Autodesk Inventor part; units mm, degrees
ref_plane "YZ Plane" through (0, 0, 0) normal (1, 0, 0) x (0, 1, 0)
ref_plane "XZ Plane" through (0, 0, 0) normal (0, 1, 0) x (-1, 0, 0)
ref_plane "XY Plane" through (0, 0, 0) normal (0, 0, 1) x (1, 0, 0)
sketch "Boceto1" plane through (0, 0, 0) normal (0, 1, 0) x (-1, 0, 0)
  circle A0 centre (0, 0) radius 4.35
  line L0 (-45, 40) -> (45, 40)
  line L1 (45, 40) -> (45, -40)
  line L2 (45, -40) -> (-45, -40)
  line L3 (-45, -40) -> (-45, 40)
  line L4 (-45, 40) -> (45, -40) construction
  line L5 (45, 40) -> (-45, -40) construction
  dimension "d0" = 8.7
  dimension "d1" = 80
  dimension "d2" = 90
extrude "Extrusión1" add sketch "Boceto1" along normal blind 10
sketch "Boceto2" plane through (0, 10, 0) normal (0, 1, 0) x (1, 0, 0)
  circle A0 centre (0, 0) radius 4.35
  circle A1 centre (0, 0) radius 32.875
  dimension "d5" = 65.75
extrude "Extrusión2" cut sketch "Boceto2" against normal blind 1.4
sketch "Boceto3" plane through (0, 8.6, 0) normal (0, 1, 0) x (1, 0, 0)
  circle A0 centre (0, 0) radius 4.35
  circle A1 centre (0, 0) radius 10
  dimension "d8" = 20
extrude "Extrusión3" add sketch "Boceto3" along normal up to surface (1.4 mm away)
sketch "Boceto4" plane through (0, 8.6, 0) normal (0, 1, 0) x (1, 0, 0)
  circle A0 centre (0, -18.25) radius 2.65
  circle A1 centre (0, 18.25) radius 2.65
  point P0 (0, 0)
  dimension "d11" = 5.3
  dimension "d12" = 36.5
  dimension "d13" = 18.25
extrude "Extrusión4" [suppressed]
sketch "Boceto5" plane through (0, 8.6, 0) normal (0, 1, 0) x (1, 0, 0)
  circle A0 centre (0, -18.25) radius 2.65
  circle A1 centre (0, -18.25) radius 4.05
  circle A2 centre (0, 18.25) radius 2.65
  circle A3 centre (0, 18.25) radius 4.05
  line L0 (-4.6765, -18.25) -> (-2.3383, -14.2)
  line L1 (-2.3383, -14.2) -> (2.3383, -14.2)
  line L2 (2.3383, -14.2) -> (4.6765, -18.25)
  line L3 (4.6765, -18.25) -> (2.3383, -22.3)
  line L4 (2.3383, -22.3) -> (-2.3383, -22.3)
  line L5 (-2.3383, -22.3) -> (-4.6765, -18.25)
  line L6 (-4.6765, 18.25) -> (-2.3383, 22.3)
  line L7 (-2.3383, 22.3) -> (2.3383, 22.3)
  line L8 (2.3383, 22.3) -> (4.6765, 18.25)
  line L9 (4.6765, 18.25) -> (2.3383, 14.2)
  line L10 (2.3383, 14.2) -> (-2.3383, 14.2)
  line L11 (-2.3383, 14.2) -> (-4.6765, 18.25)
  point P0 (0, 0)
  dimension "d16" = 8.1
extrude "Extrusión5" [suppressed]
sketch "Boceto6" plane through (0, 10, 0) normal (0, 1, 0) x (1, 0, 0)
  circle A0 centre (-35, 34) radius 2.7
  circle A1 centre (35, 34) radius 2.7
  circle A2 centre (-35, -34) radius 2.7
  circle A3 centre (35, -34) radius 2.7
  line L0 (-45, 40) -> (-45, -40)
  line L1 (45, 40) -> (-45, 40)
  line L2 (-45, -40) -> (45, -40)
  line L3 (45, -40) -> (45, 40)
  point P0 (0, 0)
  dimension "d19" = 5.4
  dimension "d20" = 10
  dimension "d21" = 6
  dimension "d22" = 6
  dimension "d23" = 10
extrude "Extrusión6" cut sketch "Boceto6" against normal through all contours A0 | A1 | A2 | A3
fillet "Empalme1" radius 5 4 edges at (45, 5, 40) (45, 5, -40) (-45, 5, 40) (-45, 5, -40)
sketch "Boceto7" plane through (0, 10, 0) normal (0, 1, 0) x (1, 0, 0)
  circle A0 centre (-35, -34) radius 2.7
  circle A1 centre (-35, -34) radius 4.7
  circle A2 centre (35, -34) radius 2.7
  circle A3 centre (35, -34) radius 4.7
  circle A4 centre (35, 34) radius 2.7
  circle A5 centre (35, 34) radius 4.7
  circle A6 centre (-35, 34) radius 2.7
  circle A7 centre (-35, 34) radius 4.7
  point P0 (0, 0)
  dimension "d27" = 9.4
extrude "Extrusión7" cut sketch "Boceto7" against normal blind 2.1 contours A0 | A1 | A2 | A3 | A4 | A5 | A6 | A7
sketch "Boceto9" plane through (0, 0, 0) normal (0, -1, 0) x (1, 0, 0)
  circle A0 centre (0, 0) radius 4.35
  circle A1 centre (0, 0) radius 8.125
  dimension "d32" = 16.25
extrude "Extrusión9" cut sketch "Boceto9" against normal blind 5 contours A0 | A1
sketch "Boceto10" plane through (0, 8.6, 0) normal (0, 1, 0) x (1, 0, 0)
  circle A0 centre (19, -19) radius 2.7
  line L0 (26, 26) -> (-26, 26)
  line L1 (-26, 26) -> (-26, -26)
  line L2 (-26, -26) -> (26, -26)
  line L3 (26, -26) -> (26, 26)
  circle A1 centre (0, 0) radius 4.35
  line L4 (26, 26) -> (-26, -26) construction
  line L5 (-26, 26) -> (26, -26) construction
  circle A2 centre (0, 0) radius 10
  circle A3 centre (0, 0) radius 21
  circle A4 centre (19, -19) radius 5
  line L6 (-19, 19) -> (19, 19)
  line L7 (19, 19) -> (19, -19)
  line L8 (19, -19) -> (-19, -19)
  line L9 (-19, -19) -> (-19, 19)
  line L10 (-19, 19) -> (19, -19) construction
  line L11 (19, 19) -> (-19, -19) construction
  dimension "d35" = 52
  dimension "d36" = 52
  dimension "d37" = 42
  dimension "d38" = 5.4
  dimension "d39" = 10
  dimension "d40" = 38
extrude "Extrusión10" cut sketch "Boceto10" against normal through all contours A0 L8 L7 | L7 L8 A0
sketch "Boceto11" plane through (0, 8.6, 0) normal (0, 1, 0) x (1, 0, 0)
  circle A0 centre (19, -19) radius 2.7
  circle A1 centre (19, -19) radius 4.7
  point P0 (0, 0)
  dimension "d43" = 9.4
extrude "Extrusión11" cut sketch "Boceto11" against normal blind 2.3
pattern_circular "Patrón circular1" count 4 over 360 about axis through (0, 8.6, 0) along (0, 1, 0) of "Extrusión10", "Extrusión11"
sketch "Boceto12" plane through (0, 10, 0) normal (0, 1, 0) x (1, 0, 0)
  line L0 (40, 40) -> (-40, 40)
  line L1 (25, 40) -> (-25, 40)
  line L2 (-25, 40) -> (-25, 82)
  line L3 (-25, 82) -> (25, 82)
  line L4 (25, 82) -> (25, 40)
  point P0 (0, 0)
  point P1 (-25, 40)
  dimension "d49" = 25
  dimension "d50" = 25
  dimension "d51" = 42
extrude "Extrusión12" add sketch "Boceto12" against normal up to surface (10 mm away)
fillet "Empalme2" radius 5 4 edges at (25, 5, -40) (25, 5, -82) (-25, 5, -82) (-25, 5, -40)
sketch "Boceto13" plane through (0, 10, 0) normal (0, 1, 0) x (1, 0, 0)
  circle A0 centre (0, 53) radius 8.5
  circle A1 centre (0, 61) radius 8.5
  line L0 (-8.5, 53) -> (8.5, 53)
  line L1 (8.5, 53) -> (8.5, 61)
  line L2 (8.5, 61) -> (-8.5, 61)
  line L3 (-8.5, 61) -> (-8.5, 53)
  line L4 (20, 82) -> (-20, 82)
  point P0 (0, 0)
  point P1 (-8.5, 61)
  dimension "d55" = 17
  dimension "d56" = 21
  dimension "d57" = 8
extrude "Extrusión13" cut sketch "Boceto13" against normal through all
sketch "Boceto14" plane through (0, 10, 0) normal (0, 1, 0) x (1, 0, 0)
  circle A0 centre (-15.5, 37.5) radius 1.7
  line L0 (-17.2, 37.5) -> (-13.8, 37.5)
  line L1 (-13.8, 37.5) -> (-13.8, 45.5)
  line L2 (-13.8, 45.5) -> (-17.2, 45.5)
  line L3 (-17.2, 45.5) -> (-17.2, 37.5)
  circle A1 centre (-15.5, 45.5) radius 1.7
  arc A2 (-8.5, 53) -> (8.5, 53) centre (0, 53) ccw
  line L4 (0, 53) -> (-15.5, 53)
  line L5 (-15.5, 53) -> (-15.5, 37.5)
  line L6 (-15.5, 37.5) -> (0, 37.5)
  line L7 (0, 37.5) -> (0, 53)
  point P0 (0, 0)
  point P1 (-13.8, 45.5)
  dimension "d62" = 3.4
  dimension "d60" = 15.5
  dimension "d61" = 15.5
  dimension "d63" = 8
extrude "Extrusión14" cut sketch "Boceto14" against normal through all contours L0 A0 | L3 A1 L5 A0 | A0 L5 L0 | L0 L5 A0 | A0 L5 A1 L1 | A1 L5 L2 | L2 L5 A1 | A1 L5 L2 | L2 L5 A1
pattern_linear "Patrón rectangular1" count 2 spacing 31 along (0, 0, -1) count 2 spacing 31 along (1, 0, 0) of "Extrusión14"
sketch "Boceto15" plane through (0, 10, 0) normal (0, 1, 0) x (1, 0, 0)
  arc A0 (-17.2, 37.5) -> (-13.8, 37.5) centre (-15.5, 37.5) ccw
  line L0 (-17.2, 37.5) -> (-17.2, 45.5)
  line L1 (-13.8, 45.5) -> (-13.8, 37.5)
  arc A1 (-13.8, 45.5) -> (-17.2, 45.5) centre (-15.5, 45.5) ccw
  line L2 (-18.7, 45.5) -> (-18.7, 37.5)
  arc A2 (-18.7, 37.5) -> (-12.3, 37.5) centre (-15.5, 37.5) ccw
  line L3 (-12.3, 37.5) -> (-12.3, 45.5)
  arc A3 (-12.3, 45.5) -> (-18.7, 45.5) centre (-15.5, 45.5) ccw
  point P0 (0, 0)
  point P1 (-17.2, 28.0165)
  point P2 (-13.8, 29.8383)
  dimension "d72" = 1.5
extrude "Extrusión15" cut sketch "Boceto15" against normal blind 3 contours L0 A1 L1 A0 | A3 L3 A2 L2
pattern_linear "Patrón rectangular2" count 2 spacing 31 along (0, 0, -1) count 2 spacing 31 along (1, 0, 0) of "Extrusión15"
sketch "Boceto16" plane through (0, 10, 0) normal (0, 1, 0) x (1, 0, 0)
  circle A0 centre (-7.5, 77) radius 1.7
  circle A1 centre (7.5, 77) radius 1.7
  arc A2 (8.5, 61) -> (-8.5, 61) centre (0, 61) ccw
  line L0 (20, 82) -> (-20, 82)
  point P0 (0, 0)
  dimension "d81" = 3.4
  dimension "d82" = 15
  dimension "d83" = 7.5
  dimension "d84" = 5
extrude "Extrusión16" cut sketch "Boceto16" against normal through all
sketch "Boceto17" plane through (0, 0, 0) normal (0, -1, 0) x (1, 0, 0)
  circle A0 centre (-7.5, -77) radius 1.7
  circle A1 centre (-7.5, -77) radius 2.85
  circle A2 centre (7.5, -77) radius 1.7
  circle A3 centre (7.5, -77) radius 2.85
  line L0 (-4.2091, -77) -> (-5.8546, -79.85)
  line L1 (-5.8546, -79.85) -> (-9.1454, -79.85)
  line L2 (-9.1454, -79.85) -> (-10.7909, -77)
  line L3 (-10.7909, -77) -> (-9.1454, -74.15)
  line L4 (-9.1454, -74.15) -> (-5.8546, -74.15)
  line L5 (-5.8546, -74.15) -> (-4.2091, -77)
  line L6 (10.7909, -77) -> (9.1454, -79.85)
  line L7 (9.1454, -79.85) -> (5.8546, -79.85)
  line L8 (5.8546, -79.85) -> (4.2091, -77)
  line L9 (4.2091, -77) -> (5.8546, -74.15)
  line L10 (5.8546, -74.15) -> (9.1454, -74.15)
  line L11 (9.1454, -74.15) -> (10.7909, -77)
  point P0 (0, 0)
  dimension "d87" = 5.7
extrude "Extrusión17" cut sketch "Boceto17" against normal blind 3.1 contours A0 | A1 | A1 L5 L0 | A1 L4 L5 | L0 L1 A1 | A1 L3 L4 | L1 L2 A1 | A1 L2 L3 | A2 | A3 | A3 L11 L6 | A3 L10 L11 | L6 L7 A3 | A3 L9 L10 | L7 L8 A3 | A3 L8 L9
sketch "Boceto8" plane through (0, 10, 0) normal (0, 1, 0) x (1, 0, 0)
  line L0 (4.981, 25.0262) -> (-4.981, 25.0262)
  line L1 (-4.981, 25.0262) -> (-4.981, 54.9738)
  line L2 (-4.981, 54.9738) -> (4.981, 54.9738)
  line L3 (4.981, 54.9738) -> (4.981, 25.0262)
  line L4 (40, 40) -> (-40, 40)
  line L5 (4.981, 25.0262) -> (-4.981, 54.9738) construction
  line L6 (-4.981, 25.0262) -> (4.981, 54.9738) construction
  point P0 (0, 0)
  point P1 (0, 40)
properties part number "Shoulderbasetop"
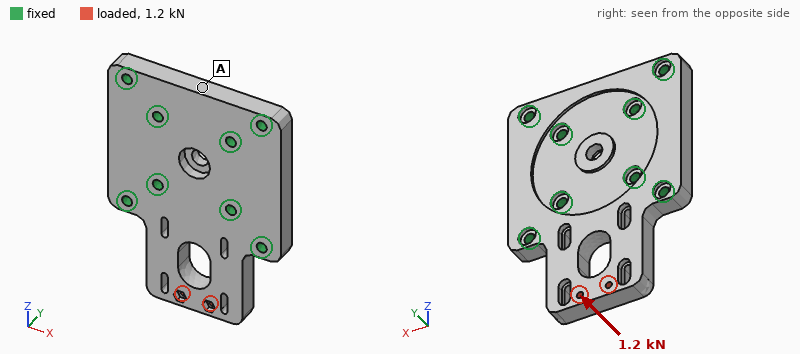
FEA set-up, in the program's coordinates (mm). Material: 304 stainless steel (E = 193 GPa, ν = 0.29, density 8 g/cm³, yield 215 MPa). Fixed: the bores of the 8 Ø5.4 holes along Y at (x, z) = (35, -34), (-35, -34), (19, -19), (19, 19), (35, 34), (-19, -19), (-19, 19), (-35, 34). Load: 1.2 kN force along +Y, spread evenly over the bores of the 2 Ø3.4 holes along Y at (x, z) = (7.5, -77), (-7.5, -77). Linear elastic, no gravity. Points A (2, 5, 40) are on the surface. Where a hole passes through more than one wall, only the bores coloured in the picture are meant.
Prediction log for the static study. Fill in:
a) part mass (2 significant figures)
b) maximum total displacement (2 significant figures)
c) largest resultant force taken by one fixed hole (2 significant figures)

630 g
0.12 mm
970 N
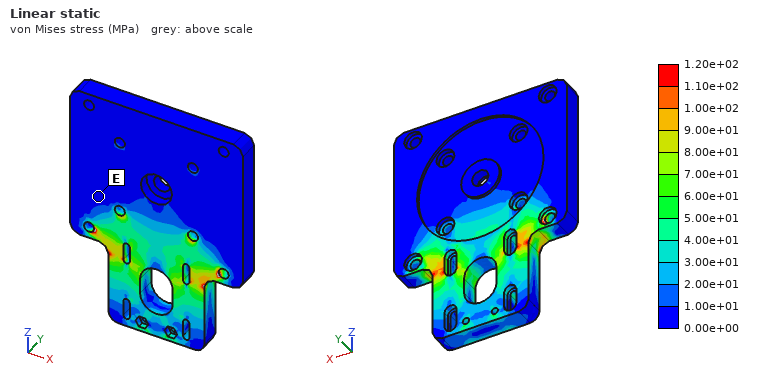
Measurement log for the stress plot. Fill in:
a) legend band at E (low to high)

0.00e+00 to 1.00e+01 MPa
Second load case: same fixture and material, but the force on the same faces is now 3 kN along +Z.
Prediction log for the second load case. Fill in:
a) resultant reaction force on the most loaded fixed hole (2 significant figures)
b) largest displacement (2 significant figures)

810 N
18 µm
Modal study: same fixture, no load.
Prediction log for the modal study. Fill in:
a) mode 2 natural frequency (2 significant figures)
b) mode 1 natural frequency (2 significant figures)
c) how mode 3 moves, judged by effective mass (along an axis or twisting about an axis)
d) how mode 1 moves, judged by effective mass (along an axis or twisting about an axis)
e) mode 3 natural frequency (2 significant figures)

5700 Hz
2400 Hz
along X
along Y
8900 Hz
